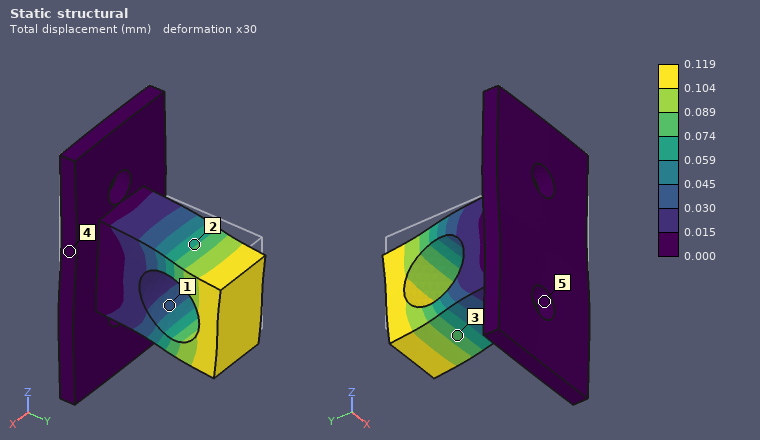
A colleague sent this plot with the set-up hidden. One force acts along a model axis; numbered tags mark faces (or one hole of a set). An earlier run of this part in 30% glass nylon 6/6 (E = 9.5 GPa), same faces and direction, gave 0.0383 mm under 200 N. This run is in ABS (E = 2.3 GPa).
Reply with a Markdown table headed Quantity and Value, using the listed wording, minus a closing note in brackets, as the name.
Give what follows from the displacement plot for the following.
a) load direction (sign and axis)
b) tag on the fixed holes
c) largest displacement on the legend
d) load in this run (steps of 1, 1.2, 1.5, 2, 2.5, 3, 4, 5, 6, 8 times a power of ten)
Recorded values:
| Quantity | Value |
|---|---|
| load direction | -Z |
| tag on the fixed holes | 5 |
| largest displacement on the legend | 0.119 mm |
| load in this run | 150 N |
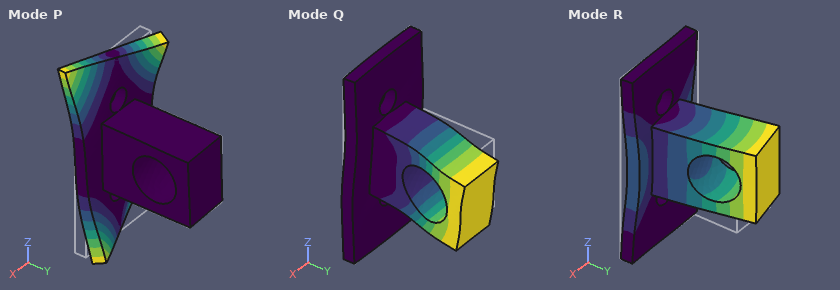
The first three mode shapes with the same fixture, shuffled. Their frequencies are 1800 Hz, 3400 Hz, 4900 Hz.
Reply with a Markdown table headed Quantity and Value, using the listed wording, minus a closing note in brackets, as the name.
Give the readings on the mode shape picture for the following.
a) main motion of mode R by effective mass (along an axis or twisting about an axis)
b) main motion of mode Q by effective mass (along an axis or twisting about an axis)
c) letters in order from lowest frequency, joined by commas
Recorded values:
| Quantity | Value |
|---|---|
| main motion of mode R by effective mass | along X |
| main motion of mode Q by effective mass | along Z |
| letters in order from lowest frequency, joined by commas | R, Q, P |
